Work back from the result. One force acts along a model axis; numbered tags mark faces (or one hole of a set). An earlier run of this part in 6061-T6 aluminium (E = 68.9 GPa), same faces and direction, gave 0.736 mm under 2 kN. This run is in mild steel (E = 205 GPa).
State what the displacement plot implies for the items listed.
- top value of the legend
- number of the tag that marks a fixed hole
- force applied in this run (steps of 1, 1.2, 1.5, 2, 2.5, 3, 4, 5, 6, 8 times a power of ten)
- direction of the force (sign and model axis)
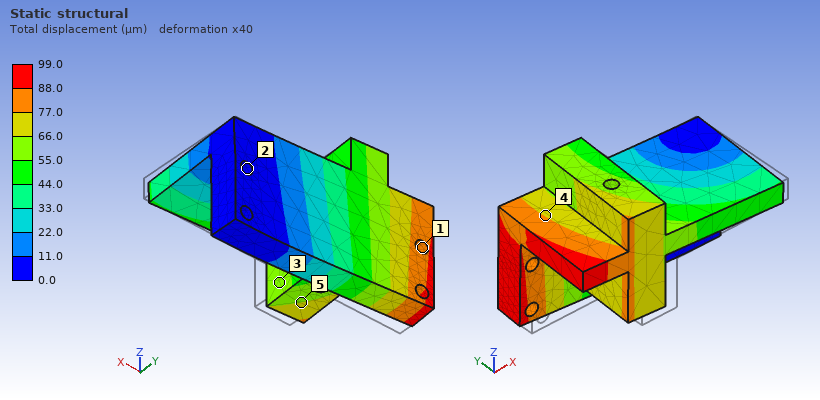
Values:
99.0 µm
2
800 N
+Y
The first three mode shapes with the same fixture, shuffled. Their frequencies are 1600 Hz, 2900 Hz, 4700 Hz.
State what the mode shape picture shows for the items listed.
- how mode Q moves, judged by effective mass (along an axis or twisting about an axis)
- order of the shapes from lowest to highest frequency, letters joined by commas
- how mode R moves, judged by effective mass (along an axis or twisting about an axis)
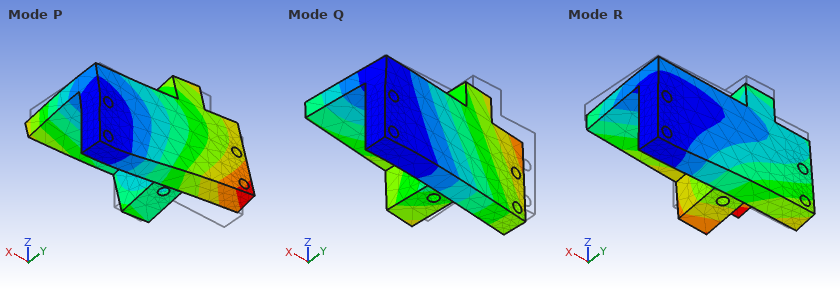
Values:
along Y
Q, R, P
along Z
